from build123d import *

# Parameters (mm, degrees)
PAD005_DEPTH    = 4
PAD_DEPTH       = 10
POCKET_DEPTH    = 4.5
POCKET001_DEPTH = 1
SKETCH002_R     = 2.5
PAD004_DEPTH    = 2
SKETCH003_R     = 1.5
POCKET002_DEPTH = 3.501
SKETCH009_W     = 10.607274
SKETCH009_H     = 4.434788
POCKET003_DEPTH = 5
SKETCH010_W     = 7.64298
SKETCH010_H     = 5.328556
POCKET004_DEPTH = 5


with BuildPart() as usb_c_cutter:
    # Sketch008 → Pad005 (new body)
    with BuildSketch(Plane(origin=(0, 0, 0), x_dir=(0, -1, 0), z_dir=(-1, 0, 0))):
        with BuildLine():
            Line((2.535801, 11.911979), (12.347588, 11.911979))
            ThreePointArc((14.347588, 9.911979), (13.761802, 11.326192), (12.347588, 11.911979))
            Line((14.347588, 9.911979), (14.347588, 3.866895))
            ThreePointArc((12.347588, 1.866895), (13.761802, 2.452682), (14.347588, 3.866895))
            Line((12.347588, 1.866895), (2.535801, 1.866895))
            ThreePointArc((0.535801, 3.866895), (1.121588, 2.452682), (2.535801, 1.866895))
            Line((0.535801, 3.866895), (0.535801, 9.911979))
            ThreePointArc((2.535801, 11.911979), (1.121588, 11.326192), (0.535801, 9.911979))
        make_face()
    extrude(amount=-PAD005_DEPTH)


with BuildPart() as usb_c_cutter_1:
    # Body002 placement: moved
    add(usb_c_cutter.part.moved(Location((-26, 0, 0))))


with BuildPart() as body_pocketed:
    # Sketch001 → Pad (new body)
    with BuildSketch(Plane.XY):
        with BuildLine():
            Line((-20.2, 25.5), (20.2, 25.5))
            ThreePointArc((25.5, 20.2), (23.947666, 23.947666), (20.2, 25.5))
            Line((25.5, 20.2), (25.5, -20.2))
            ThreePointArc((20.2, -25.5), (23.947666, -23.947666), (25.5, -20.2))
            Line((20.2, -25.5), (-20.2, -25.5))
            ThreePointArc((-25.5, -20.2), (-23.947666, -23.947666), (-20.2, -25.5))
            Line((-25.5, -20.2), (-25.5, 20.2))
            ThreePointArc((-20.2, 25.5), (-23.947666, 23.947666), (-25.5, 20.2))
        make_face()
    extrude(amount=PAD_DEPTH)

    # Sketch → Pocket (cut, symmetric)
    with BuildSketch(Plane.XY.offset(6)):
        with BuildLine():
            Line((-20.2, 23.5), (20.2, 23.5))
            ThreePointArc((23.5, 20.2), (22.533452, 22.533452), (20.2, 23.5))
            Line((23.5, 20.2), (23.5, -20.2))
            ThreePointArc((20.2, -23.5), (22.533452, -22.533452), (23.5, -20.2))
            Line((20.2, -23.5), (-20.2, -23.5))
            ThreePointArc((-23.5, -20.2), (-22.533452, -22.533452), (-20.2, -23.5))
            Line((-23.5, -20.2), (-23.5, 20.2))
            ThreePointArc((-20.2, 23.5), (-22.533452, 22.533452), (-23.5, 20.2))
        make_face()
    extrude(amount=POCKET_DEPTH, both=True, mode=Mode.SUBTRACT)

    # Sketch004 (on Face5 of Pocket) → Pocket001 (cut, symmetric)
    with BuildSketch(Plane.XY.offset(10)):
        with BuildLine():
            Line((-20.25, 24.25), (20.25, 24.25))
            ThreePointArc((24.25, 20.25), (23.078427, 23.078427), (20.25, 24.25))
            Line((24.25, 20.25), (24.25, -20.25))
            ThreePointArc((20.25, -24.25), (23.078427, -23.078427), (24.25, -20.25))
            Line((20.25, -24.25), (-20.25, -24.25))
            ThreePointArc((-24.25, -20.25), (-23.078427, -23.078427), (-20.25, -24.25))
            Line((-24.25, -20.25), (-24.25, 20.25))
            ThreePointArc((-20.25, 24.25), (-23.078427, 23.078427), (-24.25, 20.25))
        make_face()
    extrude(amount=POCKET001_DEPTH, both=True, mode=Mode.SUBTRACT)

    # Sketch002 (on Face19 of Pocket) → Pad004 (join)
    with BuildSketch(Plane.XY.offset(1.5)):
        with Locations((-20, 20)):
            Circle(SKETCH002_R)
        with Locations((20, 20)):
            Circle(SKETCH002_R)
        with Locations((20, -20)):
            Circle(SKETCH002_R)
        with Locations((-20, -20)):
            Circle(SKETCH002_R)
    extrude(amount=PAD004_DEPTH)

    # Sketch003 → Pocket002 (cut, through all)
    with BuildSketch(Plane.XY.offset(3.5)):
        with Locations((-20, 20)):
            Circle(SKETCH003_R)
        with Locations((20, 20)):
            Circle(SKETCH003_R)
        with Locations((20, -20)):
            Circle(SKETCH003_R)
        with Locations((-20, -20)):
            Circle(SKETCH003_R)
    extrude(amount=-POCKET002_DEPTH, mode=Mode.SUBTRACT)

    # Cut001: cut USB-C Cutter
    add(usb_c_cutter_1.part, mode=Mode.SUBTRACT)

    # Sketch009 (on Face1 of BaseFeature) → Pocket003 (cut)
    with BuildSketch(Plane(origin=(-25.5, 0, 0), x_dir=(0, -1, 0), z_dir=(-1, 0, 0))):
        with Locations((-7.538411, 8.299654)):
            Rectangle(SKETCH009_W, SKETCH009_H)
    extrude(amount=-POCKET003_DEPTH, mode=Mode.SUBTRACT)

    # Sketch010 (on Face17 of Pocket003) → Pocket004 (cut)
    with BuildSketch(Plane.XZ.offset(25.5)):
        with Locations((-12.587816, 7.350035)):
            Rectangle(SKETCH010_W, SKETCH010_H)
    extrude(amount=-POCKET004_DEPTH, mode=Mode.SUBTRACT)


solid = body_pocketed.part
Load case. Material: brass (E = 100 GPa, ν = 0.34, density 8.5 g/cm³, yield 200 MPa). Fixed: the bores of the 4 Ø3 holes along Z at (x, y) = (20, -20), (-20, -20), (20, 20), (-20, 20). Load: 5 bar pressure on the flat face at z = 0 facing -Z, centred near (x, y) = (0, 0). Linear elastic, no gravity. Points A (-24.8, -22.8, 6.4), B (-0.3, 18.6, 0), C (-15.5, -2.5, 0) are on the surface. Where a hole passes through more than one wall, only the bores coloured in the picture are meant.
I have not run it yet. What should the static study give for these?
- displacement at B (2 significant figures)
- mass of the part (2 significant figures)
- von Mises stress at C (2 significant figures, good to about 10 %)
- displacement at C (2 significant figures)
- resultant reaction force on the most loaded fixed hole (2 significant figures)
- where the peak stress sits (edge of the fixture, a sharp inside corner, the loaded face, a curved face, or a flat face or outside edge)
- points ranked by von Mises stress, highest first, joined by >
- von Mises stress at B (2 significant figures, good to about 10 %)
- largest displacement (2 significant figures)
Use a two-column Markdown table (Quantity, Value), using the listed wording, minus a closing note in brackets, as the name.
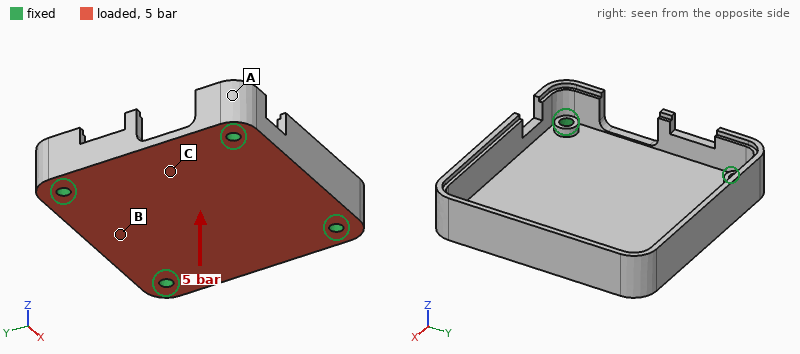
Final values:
| Quantity | Value |
|---|---|
| displacement at B | 0.052 mm |
| mass of the part | 56 g |
| von Mises stress at C | 70 MPa |
| displacement at C | 0.11 mm |
| resultant reaction force on the most loaded fixed hole | 340 N |
| where the peak stress sits | the loaded face |
| points ranked by von Mises stress, highest first, joined by > | C > B > A |
| von Mises stress at B | 31 MPa |
| largest displacement | 0.17 mm |
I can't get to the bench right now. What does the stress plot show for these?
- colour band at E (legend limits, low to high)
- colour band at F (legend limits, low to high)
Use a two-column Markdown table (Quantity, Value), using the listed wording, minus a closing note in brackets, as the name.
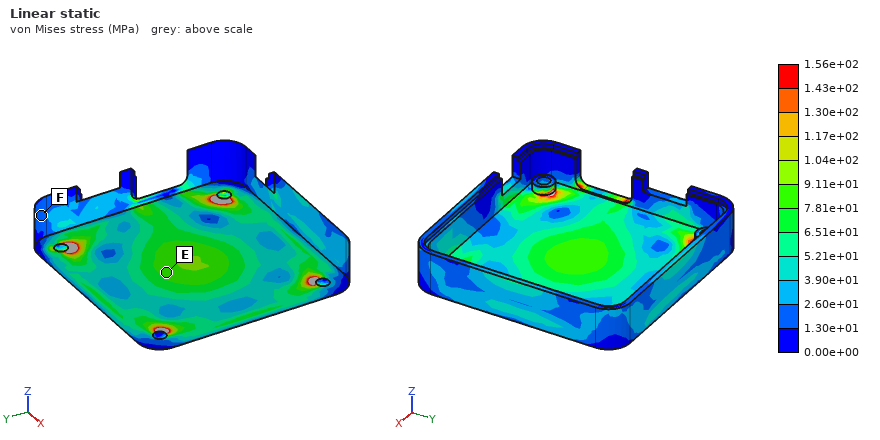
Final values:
| Quantity | Value |
|---|---|
| colour band at E | 7.81e+01 to 9.11e+01 MPa |
| colour band at F | 1.30e+01 to 2.60e+01 MPa |
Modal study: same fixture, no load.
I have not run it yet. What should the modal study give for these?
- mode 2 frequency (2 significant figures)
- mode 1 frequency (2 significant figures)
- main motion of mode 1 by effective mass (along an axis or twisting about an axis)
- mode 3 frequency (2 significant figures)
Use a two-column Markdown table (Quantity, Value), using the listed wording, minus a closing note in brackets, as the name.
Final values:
| Quantity | Value |
|---|---|
| mode 2 frequency | 5000 Hz |
| mode 1 frequency | 3000 Hz |
| main motion of mode 1 by effective mass | along Z |
| mode 3 frequency | 6000 Hz |
